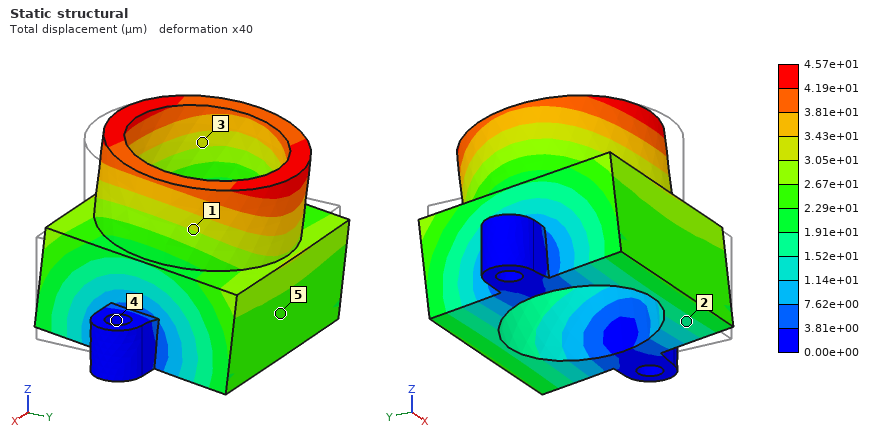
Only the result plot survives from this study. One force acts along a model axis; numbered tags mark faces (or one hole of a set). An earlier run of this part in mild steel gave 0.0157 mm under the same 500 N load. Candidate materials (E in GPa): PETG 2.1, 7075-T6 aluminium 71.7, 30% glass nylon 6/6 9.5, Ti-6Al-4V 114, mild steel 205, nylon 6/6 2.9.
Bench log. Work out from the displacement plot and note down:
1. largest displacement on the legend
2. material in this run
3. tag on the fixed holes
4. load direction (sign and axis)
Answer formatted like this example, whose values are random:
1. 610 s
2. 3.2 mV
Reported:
1. 4.57e+01 µm
2. 7075-T6 aluminium
3. 4
4. +Y
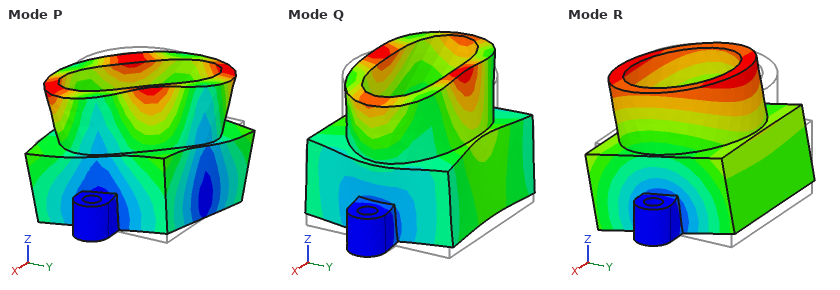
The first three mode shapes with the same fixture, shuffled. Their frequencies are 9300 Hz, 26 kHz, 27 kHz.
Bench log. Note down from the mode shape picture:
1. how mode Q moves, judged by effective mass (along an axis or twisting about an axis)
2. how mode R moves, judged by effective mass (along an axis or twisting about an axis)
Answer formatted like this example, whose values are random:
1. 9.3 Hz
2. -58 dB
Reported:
1. along Z
2. along Y
